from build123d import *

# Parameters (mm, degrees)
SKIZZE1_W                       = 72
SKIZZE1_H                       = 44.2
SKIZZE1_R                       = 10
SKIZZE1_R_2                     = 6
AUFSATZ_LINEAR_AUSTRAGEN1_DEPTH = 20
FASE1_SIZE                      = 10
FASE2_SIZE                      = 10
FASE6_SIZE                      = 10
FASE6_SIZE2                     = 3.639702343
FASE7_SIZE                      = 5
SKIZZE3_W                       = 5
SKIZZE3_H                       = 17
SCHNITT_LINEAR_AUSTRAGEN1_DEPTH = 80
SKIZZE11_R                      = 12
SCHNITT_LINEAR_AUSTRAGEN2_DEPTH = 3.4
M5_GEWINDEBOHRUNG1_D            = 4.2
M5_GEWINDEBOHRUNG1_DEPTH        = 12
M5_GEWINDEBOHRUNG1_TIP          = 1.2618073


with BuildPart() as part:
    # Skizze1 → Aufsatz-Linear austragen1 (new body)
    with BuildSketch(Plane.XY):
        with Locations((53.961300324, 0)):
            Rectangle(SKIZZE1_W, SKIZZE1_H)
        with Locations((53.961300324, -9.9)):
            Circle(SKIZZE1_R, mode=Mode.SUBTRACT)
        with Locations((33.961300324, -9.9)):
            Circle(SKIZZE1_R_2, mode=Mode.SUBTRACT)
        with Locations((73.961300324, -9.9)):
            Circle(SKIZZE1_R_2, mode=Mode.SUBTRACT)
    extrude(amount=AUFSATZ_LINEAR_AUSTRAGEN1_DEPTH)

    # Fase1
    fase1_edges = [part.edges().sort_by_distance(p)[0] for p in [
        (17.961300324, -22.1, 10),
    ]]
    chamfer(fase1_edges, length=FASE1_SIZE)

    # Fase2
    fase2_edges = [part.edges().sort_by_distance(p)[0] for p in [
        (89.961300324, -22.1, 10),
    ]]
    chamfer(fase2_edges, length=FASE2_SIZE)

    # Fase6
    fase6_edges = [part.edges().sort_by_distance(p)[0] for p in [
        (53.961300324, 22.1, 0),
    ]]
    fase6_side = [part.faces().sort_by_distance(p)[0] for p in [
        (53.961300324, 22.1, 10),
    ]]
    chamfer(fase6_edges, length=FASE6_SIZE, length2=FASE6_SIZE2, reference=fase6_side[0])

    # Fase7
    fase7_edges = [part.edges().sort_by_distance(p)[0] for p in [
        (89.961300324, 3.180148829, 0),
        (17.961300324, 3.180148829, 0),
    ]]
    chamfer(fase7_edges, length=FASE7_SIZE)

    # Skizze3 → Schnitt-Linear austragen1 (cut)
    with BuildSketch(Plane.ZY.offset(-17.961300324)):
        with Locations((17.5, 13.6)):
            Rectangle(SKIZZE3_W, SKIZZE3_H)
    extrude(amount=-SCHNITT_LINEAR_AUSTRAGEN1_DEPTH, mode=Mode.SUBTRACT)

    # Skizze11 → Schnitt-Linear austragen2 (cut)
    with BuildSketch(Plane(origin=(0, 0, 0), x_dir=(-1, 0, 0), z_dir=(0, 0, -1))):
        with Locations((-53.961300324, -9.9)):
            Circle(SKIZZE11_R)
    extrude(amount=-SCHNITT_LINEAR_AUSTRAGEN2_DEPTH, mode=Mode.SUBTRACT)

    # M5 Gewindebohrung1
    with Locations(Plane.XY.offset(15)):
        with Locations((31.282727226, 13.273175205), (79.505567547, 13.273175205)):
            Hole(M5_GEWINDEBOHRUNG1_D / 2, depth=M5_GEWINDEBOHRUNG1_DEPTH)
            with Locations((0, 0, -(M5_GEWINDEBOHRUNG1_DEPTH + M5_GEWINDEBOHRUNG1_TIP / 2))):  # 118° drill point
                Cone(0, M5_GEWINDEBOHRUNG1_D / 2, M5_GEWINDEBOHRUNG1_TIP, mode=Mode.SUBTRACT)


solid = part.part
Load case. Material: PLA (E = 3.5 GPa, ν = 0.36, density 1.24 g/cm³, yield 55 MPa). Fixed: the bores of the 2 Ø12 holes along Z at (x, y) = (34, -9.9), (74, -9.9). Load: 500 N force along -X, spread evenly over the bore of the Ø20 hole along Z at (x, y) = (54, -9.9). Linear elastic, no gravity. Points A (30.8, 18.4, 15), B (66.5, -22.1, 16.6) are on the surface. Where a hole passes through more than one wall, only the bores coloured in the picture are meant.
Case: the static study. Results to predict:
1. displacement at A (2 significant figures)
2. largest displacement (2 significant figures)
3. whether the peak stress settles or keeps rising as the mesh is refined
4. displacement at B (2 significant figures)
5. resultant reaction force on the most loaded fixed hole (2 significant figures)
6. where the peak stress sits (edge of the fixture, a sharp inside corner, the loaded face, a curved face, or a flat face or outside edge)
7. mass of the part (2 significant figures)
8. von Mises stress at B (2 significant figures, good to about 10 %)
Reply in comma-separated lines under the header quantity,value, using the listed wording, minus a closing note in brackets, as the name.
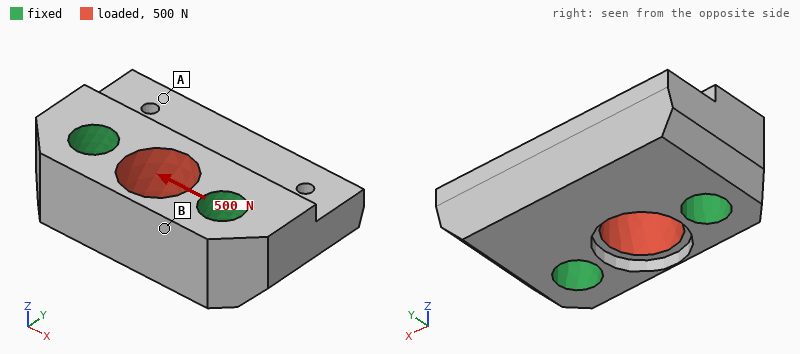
quantity,value
displacement at A,1.6 µm
largest displacement,4.6 µm
whether the peak stress settles or keeps rising as the mesh is refined,keeps rising
displacement at B,2.6 µm
resultant reaction force on the most loaded fixed hole,250 N
where the peak stress sits,a sharp inside corner
mass of the part,52 g
von Mises stress at B,0.59 MPa
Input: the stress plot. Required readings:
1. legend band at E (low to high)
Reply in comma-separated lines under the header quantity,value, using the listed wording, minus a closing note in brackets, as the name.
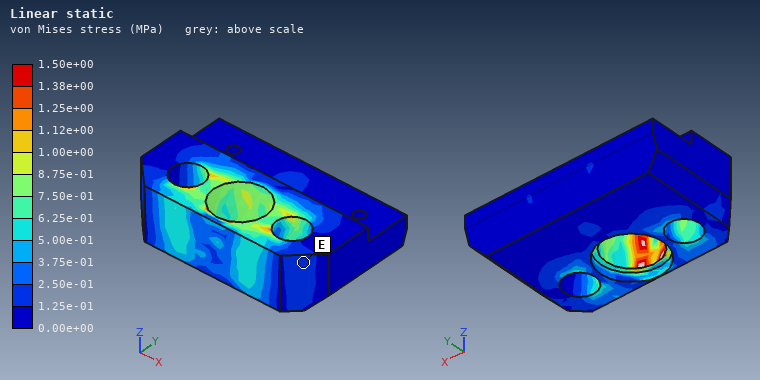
quantity,value
legend band at E,1.25e-01 to 2.50e-01 MPa
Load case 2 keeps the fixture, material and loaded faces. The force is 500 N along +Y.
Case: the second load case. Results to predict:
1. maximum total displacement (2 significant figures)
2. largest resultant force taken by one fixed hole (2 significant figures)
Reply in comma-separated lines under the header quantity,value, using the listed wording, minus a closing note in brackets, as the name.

quantity,value
maximum total displacement,18 µm
largest resultant force taken by one fixed hole,250 N
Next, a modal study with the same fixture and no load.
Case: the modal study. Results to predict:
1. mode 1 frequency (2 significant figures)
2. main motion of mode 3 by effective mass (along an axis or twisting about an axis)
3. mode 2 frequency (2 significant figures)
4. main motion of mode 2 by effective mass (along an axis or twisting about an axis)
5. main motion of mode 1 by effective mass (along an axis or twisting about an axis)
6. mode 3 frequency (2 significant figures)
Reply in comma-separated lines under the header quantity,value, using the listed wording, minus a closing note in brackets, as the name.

quantity,value
mode 1 frequency,4900 Hz
main motion of mode 3 by effective mass,along X
mode 2 frequency,6200 Hz
main motion of mode 2 by effective mass,twisting about Y
main motion of mode 1 by effective mass,along Z
mode 3 frequency,7100 Hz
